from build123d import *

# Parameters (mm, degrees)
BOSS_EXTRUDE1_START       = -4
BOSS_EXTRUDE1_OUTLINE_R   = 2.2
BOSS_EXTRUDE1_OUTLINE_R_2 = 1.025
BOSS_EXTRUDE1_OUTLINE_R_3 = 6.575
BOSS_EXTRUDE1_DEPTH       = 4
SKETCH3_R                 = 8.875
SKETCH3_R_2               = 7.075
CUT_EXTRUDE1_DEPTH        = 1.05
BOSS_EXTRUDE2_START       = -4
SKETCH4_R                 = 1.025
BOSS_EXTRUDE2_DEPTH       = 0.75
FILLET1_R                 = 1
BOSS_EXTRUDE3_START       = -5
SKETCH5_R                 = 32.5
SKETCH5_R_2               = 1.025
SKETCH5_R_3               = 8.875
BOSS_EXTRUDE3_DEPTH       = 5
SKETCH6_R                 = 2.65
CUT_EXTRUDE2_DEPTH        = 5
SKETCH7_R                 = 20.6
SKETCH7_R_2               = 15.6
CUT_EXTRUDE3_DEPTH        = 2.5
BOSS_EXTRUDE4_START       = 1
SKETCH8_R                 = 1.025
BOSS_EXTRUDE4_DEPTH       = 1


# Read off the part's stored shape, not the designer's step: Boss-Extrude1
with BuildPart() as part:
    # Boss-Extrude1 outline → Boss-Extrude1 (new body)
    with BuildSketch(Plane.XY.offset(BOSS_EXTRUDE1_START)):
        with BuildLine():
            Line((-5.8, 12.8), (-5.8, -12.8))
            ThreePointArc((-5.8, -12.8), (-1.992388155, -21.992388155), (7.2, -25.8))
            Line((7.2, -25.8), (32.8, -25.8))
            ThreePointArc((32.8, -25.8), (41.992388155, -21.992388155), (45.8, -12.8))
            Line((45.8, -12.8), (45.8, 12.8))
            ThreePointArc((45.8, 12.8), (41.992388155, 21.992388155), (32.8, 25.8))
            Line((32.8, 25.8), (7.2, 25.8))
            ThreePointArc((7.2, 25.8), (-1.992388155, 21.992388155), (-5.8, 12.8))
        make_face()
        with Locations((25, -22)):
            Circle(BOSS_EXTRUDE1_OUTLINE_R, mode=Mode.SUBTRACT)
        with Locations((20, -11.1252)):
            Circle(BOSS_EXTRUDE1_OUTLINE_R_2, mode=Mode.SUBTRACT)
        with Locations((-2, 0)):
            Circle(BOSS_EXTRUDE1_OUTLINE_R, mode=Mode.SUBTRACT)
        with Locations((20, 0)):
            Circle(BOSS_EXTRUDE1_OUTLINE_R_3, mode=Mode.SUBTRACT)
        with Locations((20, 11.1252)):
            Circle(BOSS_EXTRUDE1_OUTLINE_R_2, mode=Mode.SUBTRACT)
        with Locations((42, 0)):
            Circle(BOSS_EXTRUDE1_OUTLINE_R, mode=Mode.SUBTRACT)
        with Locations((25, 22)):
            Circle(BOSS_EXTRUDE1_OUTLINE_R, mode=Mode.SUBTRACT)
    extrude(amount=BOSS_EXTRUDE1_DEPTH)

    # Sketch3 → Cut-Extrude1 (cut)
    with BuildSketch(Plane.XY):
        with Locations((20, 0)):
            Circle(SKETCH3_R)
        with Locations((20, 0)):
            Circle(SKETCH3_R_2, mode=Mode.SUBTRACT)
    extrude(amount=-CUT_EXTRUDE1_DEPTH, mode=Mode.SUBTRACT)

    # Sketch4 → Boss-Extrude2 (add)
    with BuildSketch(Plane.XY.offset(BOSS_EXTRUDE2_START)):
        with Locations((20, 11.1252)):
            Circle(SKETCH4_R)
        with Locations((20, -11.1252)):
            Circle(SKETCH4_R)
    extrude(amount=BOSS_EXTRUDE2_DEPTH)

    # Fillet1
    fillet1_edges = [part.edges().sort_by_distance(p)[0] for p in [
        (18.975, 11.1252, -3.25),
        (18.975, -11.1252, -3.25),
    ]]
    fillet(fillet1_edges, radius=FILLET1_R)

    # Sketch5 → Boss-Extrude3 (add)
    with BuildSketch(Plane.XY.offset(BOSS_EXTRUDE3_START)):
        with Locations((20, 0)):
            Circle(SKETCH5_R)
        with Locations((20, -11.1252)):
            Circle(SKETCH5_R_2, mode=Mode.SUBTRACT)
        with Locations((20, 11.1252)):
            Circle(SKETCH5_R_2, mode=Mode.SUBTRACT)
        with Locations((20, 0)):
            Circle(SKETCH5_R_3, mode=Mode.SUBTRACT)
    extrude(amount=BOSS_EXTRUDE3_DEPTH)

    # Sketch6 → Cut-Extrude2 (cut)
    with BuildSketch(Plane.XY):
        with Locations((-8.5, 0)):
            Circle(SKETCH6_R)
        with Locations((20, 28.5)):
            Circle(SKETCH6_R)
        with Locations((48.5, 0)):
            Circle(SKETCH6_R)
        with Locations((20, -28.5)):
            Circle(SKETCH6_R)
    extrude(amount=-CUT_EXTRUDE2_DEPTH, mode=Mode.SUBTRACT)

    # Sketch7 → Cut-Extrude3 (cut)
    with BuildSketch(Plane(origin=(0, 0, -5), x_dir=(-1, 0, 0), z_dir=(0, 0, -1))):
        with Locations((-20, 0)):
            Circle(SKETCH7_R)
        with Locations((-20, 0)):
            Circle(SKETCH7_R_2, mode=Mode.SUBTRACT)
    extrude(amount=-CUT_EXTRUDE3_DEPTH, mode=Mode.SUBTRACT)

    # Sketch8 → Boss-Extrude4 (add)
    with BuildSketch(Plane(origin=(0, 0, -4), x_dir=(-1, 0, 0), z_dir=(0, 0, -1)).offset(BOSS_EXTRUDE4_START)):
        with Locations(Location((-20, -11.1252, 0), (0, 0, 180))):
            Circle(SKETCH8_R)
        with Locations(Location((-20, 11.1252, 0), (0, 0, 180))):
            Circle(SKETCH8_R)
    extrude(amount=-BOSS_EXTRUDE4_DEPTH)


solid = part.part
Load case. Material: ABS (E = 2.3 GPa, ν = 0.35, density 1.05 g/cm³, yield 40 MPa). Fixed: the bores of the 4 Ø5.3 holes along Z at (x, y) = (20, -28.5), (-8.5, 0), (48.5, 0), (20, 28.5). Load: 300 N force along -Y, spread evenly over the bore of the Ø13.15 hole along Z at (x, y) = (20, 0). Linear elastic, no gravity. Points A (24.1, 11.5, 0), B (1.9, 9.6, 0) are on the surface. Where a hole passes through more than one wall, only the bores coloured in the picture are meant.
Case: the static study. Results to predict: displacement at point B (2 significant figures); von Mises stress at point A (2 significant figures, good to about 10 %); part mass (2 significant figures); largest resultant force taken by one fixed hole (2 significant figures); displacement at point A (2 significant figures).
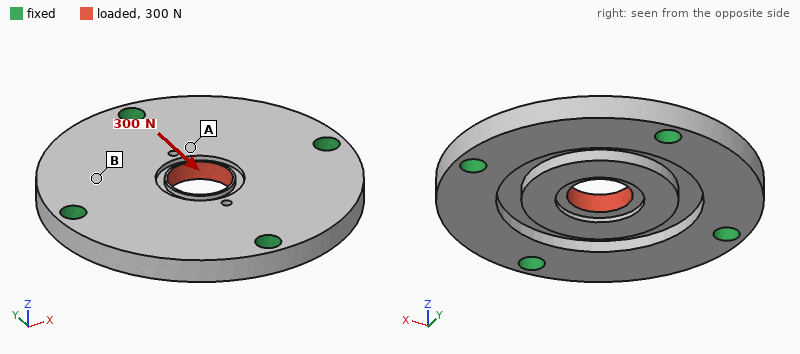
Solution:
8.9 µm
1.8 MPa
15 g
91 N
14 µm
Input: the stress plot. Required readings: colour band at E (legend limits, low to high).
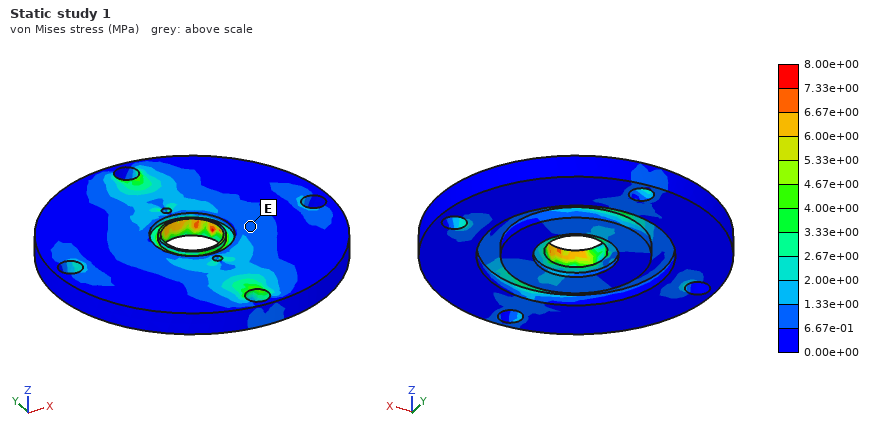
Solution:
6.67e-01 to 1.33e+00 MPa
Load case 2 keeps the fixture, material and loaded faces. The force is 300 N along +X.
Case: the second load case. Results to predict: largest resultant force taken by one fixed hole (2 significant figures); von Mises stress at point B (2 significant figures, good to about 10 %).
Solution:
92 N
0.84 MPa
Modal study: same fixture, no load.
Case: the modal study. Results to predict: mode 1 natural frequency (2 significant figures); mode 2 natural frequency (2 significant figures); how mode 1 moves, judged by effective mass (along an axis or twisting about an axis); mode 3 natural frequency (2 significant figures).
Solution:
3300 Hz
4000 Hz
along Z
4100 Hz
